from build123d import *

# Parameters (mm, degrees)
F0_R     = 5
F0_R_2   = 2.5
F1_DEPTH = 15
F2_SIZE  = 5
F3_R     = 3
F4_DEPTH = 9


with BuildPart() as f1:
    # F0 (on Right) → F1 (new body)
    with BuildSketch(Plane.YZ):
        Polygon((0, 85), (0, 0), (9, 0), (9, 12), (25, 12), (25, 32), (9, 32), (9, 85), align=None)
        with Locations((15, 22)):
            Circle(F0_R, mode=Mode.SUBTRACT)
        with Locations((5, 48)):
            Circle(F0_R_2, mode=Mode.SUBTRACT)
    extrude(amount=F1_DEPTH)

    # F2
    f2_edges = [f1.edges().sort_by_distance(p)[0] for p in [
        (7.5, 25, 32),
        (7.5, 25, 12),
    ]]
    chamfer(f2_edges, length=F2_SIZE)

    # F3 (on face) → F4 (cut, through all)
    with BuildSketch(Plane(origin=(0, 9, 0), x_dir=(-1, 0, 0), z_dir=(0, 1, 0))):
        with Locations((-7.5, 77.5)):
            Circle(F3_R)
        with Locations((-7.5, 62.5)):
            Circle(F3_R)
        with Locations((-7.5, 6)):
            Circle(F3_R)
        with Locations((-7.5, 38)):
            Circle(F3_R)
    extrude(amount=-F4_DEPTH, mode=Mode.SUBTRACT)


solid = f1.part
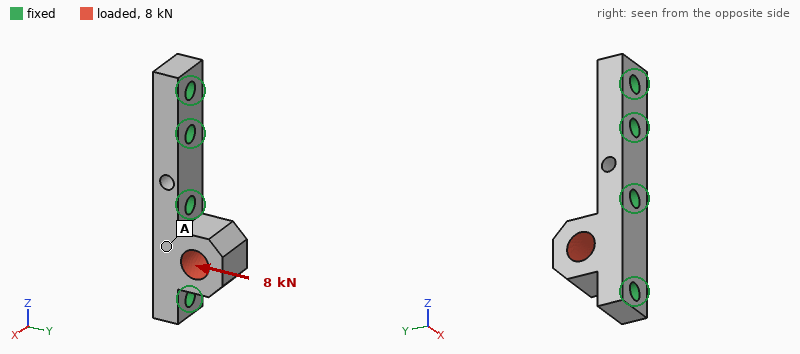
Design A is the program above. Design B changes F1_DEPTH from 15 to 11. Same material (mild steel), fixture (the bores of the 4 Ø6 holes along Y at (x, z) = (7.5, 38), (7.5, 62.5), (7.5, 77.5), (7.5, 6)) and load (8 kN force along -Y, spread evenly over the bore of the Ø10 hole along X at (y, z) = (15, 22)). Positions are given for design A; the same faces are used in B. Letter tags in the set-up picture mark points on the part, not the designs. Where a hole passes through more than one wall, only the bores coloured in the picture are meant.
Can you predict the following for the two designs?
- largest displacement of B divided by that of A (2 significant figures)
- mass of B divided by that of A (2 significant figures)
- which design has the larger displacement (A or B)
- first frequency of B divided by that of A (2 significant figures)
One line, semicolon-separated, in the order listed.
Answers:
1.5; 0.71; B; 0.90
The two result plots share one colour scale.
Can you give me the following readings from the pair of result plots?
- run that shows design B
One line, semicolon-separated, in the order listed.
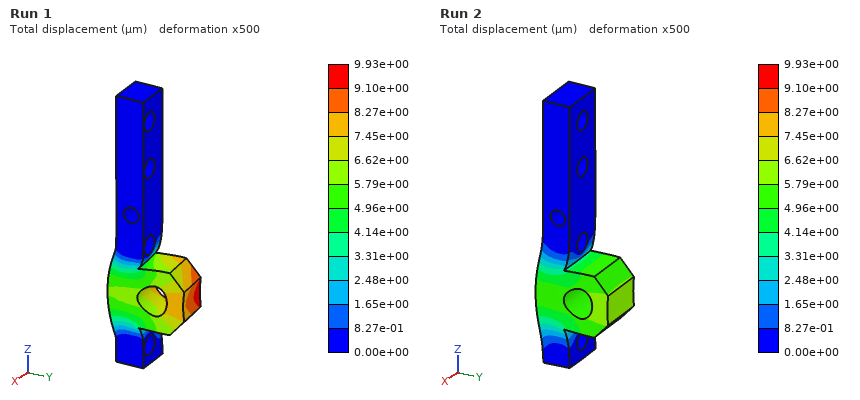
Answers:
Run 1
